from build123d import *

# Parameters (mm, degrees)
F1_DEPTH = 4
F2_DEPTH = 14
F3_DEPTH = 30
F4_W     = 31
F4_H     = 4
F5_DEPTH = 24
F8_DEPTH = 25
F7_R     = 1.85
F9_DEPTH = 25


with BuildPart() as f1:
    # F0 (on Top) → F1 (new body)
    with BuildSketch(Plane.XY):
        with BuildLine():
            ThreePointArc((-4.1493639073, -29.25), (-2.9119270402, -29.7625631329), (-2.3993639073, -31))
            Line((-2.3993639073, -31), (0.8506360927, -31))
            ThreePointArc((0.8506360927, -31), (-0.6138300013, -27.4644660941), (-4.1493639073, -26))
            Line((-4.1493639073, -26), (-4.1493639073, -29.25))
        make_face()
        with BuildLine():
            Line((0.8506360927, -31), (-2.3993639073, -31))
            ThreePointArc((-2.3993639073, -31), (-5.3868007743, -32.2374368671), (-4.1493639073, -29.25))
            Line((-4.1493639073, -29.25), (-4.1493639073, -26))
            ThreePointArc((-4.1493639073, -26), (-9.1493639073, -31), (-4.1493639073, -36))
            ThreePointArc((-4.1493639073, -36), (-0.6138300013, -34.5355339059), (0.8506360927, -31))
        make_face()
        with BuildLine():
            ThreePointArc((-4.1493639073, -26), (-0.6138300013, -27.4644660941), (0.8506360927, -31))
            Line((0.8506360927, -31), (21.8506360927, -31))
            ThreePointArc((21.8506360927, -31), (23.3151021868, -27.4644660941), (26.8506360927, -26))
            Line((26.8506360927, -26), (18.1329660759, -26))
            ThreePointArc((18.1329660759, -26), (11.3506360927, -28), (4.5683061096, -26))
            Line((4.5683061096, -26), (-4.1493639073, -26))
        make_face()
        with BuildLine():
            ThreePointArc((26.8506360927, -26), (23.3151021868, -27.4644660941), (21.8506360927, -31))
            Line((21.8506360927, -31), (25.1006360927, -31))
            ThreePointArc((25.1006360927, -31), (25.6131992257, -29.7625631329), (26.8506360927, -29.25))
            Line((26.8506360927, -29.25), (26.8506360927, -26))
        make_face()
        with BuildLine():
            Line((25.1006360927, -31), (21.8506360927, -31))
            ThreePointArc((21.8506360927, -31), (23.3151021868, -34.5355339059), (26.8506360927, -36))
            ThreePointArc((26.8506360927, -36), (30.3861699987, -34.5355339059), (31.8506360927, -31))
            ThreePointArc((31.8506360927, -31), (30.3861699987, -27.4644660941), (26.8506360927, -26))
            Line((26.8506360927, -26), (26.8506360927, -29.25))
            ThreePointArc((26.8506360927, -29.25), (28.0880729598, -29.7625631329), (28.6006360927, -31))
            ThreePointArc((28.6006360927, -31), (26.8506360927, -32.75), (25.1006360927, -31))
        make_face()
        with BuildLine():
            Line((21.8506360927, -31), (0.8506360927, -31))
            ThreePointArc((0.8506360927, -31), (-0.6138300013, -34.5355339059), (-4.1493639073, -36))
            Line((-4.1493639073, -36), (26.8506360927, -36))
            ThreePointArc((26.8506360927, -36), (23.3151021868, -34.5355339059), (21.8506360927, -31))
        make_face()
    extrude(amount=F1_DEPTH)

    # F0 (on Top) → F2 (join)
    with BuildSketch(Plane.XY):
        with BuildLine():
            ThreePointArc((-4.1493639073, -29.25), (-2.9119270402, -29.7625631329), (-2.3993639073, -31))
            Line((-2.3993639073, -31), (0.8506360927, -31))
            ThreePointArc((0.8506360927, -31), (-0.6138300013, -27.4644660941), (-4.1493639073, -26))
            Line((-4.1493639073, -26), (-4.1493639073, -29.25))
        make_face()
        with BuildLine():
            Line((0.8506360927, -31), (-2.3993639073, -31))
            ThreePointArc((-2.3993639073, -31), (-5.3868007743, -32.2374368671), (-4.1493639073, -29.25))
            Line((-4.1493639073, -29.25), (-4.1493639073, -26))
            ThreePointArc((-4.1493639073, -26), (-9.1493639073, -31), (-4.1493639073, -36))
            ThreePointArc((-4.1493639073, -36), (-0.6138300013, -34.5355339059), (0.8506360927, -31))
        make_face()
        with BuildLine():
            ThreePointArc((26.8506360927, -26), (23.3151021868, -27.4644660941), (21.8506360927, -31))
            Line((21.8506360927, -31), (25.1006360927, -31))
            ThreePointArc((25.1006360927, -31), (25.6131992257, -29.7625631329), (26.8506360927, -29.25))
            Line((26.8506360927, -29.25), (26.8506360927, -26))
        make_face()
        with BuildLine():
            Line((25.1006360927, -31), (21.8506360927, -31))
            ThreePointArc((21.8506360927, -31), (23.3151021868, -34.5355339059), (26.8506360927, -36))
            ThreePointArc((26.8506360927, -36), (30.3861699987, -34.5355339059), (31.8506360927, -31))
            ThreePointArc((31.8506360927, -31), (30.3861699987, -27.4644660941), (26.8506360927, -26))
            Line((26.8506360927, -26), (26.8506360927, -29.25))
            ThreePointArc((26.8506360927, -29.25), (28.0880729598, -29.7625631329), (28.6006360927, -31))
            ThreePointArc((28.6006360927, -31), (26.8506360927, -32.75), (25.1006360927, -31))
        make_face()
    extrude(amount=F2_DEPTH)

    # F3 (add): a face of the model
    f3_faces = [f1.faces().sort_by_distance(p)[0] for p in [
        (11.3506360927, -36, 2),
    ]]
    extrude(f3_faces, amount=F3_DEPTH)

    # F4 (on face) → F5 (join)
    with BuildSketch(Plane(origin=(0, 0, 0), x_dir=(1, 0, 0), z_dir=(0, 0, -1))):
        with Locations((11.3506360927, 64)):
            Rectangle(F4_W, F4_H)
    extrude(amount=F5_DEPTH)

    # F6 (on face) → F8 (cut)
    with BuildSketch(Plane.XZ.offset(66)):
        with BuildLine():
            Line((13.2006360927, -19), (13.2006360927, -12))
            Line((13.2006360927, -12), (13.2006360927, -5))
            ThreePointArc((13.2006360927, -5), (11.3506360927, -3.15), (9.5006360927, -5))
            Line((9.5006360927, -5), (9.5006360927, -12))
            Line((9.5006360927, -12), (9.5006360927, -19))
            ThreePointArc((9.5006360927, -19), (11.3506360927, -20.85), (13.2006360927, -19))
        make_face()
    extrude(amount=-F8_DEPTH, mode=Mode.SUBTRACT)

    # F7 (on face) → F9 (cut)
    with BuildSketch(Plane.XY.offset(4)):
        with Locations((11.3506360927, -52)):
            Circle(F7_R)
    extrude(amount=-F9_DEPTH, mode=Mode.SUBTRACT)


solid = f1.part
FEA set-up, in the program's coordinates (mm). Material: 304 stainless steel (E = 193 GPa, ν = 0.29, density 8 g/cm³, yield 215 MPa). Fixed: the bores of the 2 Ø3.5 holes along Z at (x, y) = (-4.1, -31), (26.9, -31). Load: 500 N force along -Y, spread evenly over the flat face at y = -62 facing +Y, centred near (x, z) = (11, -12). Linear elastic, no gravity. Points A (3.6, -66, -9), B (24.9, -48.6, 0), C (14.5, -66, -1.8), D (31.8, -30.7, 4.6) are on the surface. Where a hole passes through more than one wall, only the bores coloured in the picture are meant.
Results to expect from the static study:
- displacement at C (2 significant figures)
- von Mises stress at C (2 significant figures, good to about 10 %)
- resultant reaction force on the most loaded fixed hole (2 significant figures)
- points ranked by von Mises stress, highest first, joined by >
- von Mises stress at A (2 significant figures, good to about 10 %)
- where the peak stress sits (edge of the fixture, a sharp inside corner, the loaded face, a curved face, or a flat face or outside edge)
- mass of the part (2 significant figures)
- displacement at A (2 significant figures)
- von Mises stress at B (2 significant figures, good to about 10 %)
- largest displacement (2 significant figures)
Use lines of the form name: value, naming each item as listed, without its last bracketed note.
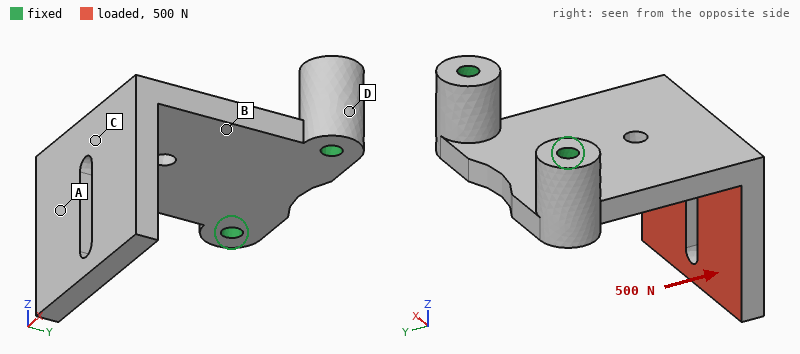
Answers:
displacement at C: 0.14 mm
von Mises stress at C: 58 MPa
resultant reaction force on the most loaded fixed hole: 270 N
points ranked by von Mises stress, highest first, joined by >: B > C > A > D
von Mises stress at A: 31 MPa
where the peak stress sits: a curved face
mass of the part: 73 g
displacement at A: 0.16 mm
von Mises stress at B: 94 MPa
largest displacement: 0.26 mm
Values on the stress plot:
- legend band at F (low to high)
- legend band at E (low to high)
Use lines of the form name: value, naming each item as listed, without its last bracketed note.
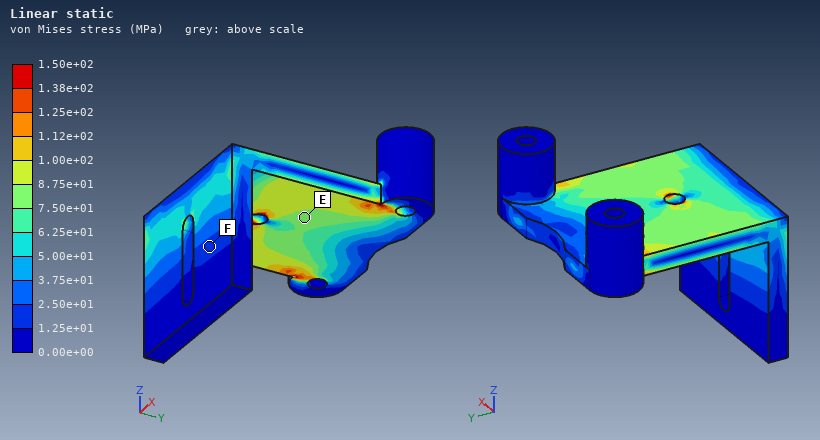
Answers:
legend band at F: 1.25e+01 to 2.50e+01 MPa
legend band at E: 7.50e+01 to 8.75e+01 MPa
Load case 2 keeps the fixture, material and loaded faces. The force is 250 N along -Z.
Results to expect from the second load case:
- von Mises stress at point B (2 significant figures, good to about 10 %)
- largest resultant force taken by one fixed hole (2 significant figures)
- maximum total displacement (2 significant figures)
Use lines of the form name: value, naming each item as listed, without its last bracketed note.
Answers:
von Mises stress at point B: 44 MPa
largest resultant force taken by one fixed hole: 130 N
maximum total displacement: 0.13 mm
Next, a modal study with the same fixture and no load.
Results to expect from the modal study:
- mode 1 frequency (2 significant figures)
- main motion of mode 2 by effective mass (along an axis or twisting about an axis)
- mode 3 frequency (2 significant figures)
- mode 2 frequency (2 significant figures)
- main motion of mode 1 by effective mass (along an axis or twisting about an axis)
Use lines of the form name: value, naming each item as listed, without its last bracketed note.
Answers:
mode 1 frequency: 1200 Hz
main motion of mode 2 by effective mass: along X
mode 3 frequency: 3700 Hz
mode 2 frequency: 2600 Hz
main motion of mode 1 by effective mass: along Z
